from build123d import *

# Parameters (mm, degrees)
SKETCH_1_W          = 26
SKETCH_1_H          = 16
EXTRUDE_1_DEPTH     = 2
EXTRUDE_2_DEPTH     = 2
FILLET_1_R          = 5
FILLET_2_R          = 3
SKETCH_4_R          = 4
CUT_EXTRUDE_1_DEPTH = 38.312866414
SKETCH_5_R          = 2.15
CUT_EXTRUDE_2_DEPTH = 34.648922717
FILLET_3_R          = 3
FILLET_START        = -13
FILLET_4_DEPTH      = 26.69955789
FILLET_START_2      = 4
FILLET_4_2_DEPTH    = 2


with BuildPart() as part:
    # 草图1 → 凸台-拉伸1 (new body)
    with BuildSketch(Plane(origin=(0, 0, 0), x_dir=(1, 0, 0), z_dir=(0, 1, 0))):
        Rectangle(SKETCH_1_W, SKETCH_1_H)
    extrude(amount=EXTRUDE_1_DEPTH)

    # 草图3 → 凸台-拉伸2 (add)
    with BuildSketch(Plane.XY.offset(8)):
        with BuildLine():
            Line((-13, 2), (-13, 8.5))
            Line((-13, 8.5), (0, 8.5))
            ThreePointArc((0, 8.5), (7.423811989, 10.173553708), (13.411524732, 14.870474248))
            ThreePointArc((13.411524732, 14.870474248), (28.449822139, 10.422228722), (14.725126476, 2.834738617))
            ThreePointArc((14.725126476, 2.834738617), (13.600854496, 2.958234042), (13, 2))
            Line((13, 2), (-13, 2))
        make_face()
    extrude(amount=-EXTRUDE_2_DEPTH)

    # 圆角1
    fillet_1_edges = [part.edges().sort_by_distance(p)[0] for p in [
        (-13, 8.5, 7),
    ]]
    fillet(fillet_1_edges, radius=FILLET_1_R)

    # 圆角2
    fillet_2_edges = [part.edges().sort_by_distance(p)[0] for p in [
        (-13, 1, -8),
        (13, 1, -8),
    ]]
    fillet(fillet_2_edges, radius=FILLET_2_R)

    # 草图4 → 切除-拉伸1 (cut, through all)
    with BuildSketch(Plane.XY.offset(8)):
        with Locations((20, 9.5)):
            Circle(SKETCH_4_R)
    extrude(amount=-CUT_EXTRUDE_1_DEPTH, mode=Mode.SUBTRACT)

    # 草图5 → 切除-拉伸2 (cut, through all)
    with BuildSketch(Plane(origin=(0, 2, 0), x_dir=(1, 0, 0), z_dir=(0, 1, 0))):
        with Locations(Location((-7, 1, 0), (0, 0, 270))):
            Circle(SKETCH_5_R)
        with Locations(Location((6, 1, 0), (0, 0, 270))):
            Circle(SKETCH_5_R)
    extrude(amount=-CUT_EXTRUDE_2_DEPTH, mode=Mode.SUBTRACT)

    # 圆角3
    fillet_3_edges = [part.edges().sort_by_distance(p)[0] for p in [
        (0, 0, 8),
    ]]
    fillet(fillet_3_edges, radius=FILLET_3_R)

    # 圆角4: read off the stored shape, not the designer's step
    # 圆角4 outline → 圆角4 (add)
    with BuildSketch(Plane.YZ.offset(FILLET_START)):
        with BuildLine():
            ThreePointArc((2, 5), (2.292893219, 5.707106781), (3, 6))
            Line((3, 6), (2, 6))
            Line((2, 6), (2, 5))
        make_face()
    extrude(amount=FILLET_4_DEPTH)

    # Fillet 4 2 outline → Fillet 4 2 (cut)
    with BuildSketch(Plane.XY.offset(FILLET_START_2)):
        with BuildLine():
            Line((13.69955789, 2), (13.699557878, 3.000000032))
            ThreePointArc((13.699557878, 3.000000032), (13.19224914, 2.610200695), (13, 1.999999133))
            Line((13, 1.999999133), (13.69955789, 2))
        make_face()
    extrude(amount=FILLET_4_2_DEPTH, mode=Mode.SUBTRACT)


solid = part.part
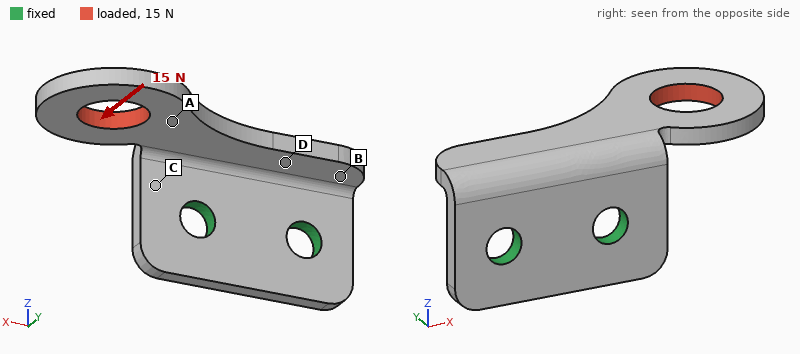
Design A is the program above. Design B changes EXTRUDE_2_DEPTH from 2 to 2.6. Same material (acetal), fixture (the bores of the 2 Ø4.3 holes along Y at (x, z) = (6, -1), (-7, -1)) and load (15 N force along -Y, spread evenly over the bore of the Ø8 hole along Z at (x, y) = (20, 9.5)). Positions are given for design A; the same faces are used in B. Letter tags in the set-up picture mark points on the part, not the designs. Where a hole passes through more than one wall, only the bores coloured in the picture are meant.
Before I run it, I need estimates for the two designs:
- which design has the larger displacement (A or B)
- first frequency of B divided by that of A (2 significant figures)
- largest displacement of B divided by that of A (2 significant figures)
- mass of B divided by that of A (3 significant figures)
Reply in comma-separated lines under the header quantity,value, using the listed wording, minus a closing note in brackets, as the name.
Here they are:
quantity,value
which design has the larger displacement,A
first frequency of B divided by that of A,1.1
largest displacement of B divided by that of A,0.77
mass of B divided by that of A,1.15
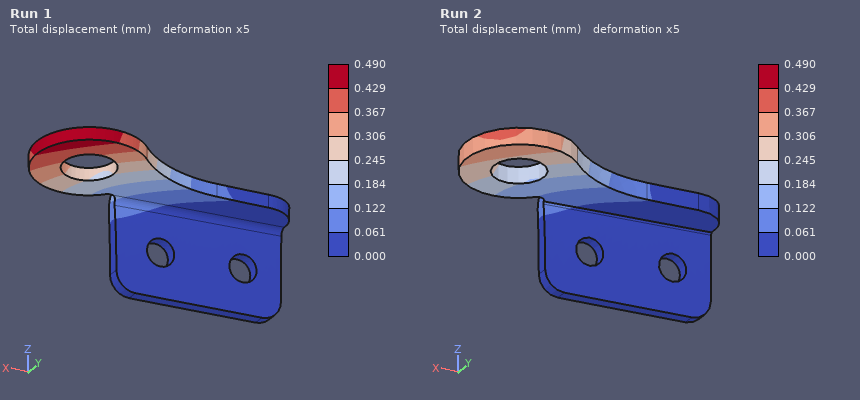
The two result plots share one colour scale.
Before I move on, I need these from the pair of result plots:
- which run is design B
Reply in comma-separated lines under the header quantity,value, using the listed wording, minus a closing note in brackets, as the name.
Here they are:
quantity,value
which run is design B,Run 2
